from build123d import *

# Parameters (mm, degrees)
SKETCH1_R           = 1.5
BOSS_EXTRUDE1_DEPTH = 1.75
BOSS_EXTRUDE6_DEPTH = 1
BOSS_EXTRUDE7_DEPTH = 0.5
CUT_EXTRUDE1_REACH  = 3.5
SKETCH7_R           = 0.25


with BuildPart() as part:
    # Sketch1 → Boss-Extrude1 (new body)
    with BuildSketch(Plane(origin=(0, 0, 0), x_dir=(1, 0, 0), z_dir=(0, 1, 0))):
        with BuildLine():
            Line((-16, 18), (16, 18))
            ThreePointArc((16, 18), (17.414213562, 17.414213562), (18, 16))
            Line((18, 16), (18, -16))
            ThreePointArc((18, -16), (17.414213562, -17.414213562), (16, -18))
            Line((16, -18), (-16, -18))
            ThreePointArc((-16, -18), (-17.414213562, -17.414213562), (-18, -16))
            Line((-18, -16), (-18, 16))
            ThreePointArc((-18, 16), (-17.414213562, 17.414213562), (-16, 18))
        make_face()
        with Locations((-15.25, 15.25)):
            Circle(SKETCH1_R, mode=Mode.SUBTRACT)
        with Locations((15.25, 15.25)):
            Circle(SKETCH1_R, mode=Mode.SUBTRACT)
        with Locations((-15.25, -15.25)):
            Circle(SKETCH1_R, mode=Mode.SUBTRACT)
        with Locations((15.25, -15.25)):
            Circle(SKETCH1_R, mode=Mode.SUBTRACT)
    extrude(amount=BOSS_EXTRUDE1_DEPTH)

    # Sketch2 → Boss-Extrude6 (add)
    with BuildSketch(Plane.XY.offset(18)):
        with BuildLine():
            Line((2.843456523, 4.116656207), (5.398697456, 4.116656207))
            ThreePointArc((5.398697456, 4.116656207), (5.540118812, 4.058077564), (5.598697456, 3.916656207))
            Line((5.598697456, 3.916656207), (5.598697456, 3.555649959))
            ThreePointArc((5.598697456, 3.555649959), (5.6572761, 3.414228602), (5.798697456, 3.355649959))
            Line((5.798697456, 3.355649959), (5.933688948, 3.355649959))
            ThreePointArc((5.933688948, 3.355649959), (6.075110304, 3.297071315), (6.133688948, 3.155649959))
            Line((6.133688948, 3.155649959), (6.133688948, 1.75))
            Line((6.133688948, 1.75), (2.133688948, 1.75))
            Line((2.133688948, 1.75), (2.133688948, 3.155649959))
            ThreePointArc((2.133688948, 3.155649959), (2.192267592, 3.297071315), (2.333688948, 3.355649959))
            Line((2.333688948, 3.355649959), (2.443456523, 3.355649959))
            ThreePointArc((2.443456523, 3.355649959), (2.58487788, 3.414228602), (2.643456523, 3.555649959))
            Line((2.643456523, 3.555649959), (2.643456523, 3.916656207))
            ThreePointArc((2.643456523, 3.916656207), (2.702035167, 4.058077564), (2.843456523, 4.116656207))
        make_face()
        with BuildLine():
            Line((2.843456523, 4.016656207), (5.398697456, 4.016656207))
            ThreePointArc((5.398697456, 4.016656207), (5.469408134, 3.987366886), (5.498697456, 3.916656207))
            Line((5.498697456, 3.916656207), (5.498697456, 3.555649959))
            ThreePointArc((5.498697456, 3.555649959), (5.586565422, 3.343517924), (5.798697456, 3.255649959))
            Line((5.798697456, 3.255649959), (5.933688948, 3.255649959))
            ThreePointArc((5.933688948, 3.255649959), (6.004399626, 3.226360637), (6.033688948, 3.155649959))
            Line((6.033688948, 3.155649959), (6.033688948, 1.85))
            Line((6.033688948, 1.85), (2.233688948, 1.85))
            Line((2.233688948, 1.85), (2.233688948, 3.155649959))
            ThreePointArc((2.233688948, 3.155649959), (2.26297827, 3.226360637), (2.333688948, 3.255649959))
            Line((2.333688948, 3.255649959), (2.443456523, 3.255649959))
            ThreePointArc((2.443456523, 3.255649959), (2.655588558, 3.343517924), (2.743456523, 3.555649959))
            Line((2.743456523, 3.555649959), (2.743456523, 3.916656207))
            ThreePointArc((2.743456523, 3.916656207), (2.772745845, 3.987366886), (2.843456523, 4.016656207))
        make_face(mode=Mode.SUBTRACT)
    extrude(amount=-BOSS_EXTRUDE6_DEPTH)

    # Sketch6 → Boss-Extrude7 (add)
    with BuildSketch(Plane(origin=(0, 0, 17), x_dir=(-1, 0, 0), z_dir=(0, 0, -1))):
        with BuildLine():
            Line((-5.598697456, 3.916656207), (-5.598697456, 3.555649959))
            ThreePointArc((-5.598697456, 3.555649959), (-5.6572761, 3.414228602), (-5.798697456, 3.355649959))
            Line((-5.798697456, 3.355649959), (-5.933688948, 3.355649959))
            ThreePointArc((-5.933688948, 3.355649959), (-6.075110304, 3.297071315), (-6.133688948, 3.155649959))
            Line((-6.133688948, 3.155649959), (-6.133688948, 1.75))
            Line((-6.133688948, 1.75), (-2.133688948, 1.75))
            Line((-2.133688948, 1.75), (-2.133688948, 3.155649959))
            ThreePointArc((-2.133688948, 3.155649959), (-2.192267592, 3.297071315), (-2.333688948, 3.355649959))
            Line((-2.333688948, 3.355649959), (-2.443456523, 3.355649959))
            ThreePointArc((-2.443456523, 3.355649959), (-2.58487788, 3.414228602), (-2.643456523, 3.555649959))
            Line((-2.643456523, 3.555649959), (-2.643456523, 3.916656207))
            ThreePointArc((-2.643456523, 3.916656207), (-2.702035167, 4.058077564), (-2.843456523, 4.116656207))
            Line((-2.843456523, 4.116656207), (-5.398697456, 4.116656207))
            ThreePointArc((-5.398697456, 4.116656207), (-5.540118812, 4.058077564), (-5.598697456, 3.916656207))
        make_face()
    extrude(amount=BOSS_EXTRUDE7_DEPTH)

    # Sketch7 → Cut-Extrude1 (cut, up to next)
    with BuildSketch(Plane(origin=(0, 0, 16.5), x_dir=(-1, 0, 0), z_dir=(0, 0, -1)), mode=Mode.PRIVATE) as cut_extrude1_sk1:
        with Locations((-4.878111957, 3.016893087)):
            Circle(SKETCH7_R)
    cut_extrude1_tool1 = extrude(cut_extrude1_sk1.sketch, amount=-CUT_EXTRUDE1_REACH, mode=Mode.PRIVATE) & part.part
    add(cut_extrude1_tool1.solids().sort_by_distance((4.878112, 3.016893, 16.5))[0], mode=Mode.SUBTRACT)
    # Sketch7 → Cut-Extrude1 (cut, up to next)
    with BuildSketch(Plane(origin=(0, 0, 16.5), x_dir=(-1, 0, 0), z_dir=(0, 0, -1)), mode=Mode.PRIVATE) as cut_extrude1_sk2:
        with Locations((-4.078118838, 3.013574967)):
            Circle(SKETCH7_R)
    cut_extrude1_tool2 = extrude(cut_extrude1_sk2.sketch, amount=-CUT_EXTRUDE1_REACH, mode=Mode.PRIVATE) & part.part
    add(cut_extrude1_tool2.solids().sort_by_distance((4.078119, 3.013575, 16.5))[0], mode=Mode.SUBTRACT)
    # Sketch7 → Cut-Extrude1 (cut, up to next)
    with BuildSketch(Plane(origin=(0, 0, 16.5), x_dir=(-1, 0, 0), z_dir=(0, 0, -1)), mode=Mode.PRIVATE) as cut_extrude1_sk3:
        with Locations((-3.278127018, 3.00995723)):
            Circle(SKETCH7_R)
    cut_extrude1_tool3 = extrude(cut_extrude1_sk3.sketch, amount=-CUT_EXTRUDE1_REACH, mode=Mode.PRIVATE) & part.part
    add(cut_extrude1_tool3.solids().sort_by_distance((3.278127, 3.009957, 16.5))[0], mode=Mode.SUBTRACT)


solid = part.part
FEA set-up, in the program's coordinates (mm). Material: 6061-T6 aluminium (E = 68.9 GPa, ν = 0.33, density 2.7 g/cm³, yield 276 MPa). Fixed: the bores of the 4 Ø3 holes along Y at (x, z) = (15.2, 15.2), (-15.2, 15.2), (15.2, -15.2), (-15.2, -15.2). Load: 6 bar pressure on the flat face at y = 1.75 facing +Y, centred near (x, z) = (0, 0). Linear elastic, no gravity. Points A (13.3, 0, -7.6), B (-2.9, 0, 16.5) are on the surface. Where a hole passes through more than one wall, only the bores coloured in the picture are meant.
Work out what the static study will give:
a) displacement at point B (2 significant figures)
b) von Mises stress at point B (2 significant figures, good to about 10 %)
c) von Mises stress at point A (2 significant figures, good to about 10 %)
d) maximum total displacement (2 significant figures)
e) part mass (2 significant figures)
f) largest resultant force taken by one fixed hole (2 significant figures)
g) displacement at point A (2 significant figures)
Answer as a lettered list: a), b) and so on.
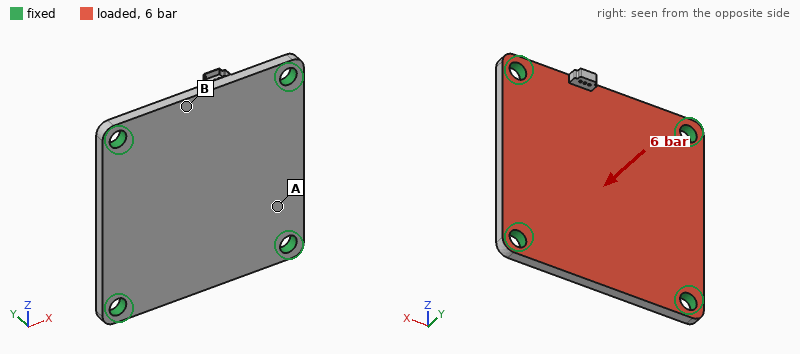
a) 42 µm
b) 48 MPa
c) 24 MPa
d) 98 µm
e) 6.0 g
f) 190 N
g) 36 µm
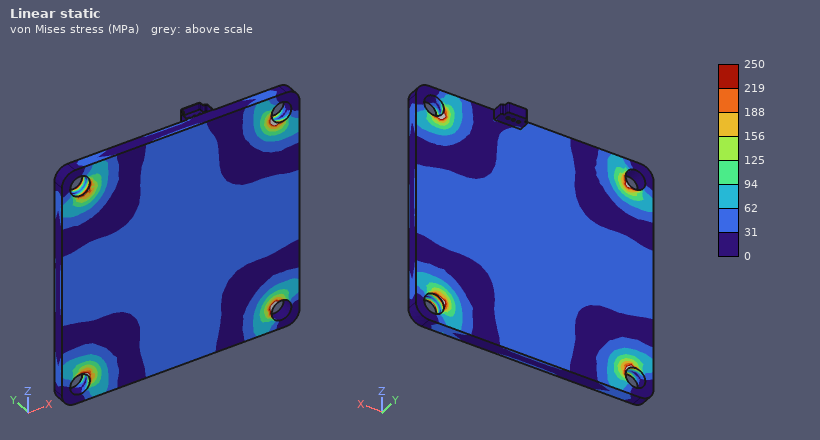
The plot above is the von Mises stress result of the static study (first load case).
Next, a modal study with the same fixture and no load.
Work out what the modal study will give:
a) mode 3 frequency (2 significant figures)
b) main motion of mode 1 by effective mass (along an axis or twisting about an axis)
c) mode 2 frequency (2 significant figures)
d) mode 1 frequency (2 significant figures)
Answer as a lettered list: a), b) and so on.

a) 12 kHz
b) along Y
c) 12 kHz
d) 7000 Hz
